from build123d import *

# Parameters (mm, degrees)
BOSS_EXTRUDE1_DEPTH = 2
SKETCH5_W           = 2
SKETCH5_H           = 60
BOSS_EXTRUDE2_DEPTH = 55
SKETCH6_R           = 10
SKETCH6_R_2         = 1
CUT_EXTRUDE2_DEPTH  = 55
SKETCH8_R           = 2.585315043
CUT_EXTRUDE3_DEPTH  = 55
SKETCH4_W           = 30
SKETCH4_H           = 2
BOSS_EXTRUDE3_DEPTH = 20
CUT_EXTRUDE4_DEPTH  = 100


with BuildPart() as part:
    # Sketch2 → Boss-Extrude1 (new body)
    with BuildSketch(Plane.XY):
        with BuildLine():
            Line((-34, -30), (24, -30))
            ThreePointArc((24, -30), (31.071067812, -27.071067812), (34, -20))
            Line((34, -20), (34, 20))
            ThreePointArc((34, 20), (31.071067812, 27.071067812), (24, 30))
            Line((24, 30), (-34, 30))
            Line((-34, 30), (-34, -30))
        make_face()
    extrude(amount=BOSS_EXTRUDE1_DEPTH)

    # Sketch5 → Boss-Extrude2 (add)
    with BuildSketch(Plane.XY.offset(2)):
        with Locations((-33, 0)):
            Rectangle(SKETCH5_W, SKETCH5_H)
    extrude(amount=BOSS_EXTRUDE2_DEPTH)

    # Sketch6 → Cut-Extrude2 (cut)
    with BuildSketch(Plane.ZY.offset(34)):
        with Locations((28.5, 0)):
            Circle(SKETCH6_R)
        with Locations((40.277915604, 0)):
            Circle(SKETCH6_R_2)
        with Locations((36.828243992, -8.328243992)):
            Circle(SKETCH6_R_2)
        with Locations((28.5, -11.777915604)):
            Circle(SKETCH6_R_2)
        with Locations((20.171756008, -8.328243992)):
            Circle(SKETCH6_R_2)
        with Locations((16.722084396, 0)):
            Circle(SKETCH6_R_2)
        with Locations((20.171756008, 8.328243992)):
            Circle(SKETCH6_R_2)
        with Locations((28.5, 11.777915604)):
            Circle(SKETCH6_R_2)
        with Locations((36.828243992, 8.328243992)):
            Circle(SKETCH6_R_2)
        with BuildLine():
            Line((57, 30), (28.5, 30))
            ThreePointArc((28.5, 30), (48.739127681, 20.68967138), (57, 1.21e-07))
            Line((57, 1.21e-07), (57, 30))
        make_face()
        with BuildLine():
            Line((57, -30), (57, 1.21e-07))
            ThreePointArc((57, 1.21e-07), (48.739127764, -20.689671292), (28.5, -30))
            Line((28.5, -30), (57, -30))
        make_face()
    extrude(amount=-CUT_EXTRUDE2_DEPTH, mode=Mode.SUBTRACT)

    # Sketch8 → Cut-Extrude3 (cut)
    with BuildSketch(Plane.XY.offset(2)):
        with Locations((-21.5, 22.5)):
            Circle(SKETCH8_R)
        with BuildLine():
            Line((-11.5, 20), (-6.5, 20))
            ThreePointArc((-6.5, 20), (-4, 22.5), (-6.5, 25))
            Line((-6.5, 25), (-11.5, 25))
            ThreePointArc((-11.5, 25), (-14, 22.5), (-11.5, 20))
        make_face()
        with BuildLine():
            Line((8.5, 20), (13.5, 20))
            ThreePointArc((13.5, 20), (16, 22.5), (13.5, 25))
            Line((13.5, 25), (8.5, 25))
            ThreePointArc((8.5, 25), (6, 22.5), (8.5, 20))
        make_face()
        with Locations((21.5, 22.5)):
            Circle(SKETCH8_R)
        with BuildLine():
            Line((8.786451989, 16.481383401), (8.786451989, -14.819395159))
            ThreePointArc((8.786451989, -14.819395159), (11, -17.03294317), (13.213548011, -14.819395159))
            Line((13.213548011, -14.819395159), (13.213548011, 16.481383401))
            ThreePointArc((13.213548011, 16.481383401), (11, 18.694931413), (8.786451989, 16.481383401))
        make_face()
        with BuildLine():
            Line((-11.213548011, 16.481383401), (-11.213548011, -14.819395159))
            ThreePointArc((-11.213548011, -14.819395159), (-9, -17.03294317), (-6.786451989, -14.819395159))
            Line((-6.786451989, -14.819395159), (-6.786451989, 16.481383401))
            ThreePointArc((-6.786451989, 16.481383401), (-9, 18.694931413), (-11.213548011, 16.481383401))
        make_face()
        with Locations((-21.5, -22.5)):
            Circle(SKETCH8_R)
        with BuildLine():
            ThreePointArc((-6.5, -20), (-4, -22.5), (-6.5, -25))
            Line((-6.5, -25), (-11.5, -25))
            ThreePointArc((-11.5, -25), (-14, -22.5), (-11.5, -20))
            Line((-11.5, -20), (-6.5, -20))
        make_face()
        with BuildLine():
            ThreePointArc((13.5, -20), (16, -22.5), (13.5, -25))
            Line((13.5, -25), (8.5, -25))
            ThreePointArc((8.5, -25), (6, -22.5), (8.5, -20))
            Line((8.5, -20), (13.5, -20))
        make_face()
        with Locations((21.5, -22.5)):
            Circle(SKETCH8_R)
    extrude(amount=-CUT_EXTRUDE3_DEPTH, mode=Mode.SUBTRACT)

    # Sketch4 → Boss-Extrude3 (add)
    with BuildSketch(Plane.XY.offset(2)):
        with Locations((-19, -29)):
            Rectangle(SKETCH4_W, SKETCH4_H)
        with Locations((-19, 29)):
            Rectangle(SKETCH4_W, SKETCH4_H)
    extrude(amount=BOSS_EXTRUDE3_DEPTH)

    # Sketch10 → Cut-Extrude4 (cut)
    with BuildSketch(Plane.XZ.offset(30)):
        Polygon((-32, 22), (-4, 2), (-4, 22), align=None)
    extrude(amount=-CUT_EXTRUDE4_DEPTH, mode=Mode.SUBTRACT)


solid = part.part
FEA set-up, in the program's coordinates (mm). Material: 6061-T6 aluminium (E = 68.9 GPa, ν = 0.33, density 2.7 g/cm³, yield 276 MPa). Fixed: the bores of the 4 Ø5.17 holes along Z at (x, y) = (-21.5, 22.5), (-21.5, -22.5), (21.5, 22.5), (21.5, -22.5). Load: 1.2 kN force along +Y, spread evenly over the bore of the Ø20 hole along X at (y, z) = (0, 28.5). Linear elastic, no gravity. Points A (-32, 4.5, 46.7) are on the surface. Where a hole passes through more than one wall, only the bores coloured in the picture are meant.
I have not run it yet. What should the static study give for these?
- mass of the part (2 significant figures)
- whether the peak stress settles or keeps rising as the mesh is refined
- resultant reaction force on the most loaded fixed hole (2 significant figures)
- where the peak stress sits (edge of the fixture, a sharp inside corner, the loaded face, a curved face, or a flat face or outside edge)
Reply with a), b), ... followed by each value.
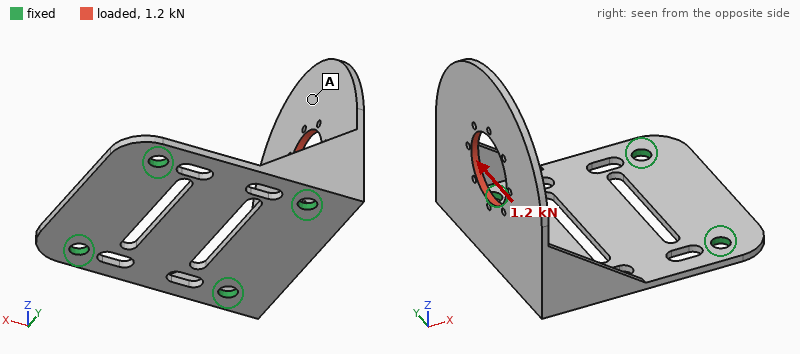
a) 36 g
b) keeps rising
c) 970 N
d) edge of the fixture
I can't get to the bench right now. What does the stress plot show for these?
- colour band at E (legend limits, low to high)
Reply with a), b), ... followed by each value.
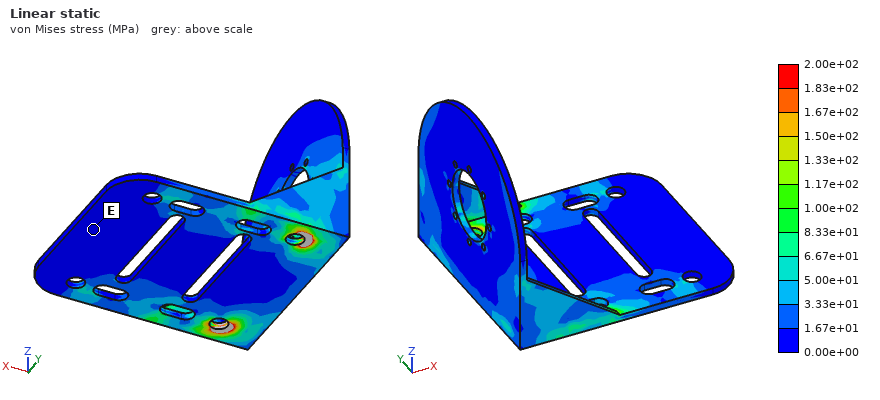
a) 0.00e+00 to 1.67e+01 MPa
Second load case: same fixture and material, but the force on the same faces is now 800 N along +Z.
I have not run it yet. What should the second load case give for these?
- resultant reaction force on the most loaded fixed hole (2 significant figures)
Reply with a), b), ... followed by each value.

a) 430 N
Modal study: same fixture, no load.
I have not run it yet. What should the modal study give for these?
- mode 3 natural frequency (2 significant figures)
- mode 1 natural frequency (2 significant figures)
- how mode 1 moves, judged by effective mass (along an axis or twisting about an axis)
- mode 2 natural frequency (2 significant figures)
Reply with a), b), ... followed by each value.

a) 3100 Hz
b) 820 Hz
c) along X
d) 2100 Hz
